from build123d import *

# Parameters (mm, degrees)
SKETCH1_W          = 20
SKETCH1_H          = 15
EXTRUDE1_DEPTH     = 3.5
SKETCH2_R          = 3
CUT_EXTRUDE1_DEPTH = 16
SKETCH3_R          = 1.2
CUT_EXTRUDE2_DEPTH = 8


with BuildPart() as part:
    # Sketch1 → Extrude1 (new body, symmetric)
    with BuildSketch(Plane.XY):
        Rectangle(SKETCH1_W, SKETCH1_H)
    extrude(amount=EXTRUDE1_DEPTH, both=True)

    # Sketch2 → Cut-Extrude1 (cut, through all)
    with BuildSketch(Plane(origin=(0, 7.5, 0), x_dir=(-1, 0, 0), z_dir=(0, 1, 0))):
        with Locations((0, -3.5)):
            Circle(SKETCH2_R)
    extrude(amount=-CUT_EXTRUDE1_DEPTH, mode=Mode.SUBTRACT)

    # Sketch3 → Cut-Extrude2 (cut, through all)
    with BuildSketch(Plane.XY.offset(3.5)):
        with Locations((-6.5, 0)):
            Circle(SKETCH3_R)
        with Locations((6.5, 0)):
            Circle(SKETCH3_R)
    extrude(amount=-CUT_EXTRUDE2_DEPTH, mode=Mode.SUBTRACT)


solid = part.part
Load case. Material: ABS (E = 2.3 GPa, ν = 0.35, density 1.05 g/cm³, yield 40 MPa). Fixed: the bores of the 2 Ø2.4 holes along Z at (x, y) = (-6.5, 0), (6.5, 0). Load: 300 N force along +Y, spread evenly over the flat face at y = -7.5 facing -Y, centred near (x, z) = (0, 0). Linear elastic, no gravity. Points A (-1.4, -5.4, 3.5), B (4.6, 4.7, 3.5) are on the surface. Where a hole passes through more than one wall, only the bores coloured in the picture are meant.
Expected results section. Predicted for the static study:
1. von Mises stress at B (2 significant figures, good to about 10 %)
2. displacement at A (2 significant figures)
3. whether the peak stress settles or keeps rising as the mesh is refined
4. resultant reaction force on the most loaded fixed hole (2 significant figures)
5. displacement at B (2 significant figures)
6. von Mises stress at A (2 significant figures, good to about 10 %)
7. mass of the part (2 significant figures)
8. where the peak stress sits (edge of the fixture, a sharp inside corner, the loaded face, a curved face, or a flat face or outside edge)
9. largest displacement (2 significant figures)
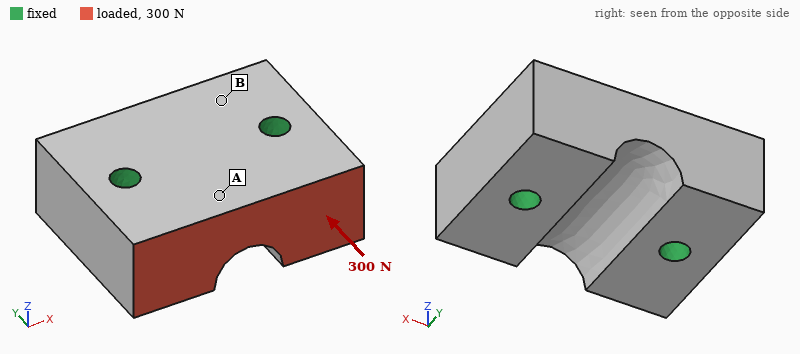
0.87 MPa
9.4 µm
keeps rising
150 N
2.7 µm
2.0 MPa
1.9 g
edge of the fixture
12 µm
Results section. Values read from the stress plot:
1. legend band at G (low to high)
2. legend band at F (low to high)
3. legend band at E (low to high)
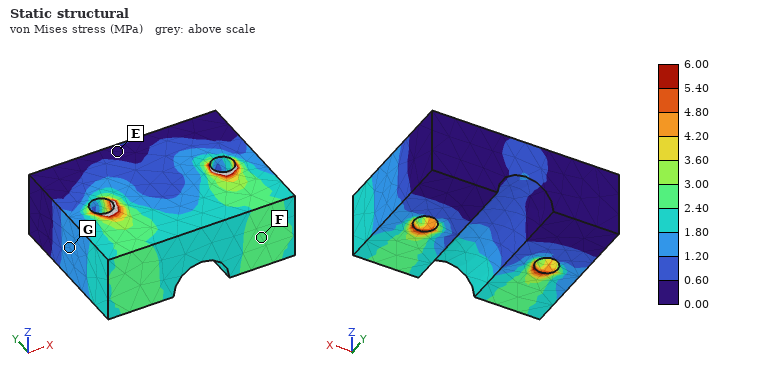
1.20 to 1.80 MPa
2.40 to 3.00 MPa
0.00 to 0.60 MPa
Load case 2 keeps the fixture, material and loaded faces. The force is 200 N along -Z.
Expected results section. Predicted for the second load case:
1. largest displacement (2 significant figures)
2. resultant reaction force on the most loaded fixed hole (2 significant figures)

55 µm
100 N
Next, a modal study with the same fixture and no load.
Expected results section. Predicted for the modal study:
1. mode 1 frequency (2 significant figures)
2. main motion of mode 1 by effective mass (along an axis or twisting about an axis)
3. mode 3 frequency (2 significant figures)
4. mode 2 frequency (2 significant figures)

17 kHz
twisting about X
21 kHz
20 kHz
